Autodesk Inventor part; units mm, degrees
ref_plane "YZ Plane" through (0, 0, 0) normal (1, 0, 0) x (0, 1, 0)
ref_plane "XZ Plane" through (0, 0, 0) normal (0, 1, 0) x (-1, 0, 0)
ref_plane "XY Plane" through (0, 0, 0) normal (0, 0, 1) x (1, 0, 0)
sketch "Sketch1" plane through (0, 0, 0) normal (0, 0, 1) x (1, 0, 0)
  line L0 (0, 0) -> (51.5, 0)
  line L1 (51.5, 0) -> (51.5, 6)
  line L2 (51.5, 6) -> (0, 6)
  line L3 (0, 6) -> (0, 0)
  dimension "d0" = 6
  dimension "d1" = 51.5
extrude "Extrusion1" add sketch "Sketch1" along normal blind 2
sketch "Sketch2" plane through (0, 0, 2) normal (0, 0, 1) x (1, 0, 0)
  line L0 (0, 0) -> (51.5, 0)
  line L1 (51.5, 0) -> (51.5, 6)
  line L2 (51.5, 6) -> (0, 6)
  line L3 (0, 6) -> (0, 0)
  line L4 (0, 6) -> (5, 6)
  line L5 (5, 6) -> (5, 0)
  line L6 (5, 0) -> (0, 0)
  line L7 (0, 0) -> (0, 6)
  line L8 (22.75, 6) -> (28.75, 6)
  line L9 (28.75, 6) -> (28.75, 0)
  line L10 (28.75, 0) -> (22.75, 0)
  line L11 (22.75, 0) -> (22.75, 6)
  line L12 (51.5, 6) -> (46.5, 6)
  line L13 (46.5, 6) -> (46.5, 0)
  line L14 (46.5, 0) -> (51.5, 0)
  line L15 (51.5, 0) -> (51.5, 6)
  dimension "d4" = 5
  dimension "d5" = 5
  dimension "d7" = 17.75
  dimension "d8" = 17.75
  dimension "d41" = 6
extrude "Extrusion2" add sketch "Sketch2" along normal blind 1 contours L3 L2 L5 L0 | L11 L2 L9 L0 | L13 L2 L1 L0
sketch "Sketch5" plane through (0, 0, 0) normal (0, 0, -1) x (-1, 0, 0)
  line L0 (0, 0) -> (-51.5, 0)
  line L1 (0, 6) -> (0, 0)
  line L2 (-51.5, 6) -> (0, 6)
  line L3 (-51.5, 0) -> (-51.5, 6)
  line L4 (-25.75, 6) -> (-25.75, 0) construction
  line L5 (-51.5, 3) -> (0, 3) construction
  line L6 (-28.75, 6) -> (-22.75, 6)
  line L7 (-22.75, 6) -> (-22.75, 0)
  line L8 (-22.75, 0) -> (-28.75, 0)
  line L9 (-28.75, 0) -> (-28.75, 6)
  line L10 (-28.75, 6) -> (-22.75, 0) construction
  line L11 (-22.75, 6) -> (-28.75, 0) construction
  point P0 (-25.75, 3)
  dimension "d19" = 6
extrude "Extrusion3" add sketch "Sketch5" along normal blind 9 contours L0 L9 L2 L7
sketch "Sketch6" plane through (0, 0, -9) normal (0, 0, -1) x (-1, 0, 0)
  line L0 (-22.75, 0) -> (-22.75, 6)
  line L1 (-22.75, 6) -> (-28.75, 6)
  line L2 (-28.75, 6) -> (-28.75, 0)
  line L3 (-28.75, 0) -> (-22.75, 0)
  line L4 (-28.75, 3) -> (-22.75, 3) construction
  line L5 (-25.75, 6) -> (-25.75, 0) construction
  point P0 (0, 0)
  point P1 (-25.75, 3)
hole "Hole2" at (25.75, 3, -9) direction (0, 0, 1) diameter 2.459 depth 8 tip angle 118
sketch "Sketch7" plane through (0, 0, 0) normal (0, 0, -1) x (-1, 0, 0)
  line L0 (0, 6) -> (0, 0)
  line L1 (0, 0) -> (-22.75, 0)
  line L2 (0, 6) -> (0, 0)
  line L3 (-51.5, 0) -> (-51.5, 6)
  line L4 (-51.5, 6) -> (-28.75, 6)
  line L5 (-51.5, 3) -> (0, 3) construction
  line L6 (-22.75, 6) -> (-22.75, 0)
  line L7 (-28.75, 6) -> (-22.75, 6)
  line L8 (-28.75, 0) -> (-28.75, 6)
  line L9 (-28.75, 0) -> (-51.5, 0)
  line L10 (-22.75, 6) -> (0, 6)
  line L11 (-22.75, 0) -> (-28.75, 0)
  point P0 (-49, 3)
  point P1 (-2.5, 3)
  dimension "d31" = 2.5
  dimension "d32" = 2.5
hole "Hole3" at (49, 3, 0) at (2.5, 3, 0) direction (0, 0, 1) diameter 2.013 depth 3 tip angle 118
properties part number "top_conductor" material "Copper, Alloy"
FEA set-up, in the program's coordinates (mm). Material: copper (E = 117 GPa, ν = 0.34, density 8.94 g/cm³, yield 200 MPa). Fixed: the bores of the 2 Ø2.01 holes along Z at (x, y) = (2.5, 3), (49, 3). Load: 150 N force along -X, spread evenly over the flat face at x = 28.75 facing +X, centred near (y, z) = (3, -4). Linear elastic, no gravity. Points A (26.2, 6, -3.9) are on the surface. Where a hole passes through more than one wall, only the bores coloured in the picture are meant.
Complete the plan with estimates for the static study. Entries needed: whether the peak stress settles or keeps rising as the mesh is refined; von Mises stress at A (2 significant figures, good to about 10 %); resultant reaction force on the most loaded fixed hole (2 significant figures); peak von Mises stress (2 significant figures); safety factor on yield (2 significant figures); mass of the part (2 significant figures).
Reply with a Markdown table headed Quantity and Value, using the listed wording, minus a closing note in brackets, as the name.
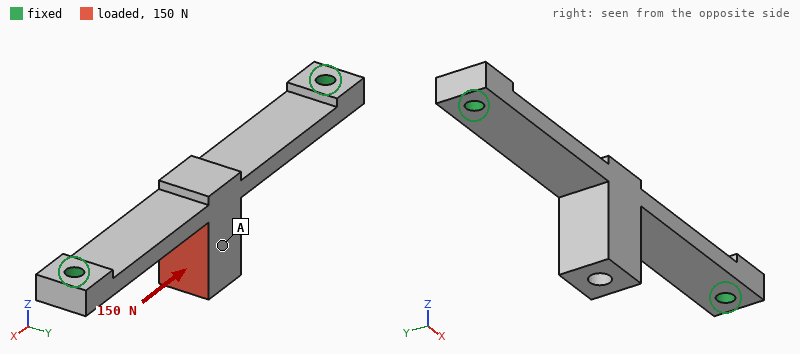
| Quantity | Value |
|---|---|
| whether the peak stress settles or keeps rising as the mesh is refined | settles |
| von Mises stress at A | 9.6 MPa |
| resultant reaction force on the most loaded fixed hole | 80 N |
| peak von Mises stress | 78 MPa |
| safety factor on yield | 2.6 |
| mass of the part | 8.8 g |
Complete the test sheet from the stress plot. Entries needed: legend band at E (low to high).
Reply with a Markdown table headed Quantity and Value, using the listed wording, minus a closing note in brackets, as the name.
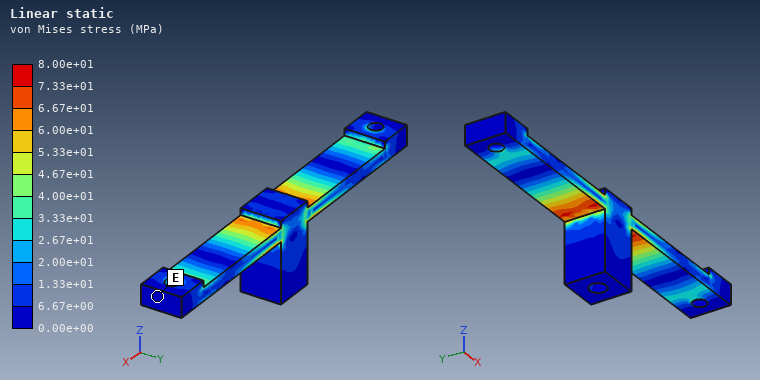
| Quantity | Value |
|---|---|
| legend band at E | 0.00e+00 to 6.67e+00 MPa |
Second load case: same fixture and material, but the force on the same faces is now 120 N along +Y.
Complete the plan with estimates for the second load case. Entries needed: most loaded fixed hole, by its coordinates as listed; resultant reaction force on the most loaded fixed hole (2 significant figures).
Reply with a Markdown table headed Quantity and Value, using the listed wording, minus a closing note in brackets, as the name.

| Quantity | Value |
|---|---|
| most loaded fixed hole, by its coordinates as listed | (49, 3) |
| resultant reaction force on the most loaded fixed hole | 71 N |
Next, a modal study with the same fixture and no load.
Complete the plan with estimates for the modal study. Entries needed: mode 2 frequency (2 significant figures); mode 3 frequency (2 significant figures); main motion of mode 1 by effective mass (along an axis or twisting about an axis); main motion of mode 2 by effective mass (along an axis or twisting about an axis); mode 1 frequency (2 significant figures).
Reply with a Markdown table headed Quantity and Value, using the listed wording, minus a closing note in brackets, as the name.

| Quantity | Value |
|---|---|
| mode 2 frequency | 3500 Hz |
| mode 3 frequency | 6500 Hz |
| main motion of mode 1 by effective mass | along Z |
| main motion of mode 2 by effective mass | along Y |
| mode 1 frequency | 2700 Hz |
